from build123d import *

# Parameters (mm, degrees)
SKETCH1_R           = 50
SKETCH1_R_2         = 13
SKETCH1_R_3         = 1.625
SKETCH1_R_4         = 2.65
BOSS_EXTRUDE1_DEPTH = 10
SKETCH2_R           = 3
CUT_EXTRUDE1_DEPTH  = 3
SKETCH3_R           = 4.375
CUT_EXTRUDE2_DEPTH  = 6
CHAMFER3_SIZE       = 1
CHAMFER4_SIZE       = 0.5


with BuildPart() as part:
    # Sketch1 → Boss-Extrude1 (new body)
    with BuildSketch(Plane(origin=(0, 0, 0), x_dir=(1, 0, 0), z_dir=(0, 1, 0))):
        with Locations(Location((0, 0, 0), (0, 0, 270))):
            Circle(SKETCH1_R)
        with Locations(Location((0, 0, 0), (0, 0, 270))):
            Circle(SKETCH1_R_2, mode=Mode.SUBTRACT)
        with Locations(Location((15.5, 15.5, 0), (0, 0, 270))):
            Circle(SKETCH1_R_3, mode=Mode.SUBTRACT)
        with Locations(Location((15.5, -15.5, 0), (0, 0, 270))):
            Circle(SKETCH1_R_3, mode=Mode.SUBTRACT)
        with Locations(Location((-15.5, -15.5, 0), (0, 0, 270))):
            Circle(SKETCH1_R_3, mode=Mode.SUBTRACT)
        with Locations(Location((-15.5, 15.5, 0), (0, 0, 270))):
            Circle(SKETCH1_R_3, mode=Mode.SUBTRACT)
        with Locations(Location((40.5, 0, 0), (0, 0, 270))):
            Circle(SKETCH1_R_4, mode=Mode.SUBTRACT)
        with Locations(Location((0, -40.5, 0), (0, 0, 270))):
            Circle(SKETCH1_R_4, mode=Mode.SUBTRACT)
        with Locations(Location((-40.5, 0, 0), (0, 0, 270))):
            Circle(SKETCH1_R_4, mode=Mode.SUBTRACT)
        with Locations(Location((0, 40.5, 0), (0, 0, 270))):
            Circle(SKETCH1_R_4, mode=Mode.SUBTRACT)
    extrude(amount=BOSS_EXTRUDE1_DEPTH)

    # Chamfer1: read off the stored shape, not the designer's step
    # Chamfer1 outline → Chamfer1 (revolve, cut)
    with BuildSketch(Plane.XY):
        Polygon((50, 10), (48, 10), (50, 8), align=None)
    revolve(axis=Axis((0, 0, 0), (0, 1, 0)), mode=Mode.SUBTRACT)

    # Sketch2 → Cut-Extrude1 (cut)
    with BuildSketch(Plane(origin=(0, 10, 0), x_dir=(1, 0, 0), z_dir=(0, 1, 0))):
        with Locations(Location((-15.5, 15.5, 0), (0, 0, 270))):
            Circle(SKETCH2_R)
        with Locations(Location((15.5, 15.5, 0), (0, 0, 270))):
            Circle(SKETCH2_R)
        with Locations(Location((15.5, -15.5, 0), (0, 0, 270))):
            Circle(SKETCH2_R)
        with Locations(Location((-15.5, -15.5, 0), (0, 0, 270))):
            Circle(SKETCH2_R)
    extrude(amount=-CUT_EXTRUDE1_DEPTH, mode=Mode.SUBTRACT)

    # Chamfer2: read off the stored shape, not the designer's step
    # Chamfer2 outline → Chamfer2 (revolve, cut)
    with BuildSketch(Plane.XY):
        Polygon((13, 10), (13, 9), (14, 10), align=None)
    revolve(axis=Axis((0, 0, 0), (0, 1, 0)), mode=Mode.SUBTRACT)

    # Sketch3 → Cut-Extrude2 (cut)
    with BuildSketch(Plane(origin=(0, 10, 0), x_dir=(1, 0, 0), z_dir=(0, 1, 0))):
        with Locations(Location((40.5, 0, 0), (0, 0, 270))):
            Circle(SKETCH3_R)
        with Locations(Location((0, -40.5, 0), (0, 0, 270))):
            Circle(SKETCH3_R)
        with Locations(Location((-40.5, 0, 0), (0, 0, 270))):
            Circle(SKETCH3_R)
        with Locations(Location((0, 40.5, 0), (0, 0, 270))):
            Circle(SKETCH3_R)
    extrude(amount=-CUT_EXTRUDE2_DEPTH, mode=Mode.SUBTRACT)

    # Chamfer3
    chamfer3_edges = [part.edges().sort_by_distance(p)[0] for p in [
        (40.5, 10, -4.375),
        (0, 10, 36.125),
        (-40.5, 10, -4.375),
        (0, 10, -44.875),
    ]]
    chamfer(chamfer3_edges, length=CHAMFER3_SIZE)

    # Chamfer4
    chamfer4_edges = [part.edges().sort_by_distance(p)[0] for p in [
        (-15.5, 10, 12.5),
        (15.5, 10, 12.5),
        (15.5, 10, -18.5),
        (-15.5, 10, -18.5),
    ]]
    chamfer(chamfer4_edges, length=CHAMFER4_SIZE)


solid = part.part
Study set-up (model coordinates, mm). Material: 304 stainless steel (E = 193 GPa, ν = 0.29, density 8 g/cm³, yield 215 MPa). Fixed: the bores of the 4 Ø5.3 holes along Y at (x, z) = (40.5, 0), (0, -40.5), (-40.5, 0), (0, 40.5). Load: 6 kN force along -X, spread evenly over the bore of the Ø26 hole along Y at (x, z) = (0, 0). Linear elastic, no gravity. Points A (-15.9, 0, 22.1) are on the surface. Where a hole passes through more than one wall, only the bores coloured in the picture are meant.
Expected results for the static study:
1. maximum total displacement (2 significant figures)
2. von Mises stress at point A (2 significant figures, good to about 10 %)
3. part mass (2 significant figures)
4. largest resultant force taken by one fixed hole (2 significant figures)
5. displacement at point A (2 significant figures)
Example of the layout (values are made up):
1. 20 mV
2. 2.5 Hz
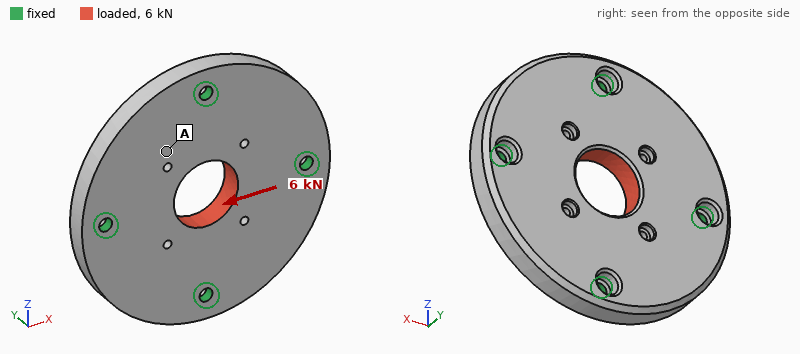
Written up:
1. 2.1 µm
2. 5.6 MPa
3. 560 g
4. 1.8 kN
5. 1.3 µm
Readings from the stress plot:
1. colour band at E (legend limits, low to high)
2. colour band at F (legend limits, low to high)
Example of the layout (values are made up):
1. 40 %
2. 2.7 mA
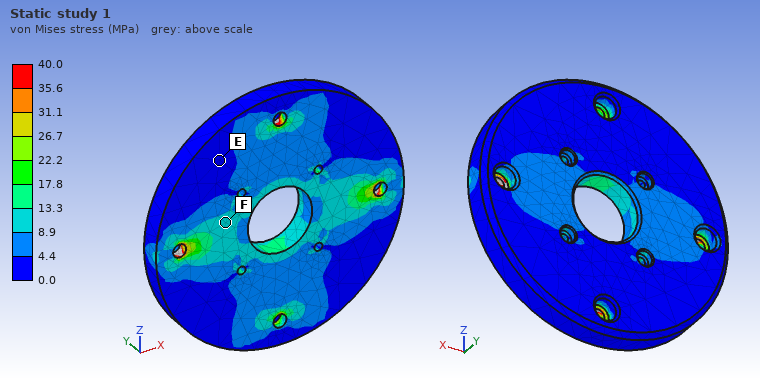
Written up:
1. 0.0 to 4.4 MPa
2. 8.9 to 13.3 MPa
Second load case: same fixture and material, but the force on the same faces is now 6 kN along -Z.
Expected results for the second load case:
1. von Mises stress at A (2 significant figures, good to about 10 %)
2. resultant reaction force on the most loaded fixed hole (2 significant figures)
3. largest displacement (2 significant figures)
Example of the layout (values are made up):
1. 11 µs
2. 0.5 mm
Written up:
1. 5.1 MPa
2. 1.8 kN
3. 2.1 µm
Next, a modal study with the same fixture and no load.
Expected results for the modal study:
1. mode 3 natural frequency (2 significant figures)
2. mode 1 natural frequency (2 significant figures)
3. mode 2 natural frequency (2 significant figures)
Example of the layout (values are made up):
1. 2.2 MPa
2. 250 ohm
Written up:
1. 8000 Hz
2. 6700 Hz
3. 7800 Hz
